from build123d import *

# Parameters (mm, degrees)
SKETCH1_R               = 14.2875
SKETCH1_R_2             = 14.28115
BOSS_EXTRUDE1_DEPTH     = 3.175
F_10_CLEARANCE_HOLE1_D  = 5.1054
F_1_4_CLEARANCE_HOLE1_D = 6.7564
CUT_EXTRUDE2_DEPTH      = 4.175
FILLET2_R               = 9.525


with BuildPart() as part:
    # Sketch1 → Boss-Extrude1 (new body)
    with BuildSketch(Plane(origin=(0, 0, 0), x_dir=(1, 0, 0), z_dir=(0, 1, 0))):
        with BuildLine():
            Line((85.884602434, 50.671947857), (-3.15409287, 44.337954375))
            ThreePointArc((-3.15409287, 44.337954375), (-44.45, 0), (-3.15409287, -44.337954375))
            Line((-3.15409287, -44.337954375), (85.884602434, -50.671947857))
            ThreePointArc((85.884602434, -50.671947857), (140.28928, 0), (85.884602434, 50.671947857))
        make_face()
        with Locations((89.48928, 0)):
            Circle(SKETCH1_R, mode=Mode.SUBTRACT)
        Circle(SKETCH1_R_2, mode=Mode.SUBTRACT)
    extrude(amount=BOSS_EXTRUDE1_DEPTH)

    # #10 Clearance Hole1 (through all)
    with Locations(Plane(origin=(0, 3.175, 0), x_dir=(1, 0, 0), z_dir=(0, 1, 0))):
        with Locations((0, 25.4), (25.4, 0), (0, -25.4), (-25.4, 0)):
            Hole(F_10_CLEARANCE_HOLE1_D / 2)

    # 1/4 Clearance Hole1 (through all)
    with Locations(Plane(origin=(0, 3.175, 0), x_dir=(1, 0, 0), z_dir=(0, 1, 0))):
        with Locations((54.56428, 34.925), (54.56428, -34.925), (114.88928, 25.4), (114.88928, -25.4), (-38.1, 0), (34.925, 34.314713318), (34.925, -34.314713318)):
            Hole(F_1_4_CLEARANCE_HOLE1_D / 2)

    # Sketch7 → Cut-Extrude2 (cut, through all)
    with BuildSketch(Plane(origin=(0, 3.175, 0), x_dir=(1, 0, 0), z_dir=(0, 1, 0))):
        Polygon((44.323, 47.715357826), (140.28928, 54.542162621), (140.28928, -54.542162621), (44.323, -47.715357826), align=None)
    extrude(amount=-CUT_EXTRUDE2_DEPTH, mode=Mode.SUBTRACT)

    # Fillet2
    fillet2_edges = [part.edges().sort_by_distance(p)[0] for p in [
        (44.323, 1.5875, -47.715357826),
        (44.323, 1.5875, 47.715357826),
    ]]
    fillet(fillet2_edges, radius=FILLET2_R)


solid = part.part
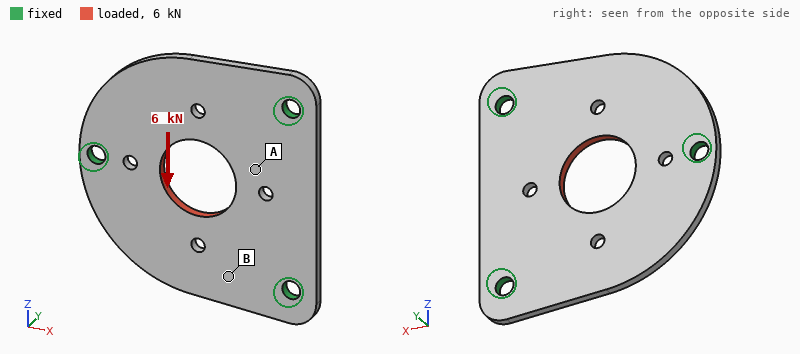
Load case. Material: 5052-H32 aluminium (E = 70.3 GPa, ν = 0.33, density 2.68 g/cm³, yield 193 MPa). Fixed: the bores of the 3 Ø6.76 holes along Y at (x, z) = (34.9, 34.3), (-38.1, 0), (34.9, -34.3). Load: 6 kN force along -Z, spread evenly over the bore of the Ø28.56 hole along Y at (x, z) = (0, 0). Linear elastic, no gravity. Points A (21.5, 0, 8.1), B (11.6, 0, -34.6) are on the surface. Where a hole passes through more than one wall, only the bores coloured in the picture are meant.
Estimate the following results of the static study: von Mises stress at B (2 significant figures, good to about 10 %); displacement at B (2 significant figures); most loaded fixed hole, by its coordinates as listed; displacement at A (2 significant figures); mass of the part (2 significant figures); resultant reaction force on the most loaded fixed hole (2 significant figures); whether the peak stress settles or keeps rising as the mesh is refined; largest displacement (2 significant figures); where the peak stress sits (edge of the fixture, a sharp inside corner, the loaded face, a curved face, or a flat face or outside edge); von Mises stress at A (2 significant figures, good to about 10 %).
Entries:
15 MPa
14 µm
(-38.1, 0)
12 µm
54 g
2.6 kN
keeps rising
25 µm
edge of the fixture
31 MPa
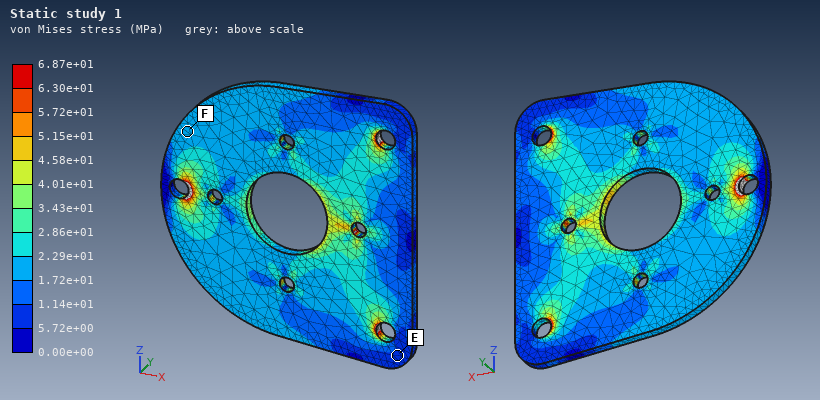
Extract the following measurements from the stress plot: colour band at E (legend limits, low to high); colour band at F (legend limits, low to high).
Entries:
5.72e+00 to 1.14e+01 MPa
1.72e+01 to 2.29e+01 MPa
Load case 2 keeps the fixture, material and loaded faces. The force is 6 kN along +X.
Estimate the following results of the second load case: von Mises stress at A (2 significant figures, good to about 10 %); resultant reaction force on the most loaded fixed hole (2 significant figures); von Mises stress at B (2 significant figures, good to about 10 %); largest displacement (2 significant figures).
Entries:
20 MPa
2.1 kN
13 MPa
22 µm
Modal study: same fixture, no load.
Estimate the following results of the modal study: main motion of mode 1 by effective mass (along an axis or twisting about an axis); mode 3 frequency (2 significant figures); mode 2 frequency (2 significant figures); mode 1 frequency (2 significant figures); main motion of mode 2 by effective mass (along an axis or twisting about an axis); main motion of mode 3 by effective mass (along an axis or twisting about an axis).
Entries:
twisting about X
3300 Hz
2200 Hz
2100 Hz
along Y
along Y
